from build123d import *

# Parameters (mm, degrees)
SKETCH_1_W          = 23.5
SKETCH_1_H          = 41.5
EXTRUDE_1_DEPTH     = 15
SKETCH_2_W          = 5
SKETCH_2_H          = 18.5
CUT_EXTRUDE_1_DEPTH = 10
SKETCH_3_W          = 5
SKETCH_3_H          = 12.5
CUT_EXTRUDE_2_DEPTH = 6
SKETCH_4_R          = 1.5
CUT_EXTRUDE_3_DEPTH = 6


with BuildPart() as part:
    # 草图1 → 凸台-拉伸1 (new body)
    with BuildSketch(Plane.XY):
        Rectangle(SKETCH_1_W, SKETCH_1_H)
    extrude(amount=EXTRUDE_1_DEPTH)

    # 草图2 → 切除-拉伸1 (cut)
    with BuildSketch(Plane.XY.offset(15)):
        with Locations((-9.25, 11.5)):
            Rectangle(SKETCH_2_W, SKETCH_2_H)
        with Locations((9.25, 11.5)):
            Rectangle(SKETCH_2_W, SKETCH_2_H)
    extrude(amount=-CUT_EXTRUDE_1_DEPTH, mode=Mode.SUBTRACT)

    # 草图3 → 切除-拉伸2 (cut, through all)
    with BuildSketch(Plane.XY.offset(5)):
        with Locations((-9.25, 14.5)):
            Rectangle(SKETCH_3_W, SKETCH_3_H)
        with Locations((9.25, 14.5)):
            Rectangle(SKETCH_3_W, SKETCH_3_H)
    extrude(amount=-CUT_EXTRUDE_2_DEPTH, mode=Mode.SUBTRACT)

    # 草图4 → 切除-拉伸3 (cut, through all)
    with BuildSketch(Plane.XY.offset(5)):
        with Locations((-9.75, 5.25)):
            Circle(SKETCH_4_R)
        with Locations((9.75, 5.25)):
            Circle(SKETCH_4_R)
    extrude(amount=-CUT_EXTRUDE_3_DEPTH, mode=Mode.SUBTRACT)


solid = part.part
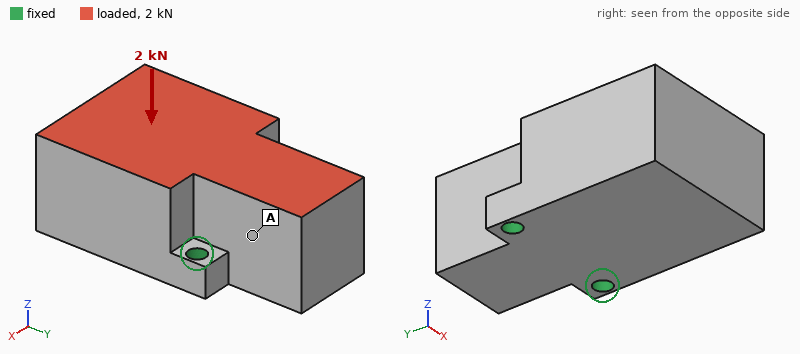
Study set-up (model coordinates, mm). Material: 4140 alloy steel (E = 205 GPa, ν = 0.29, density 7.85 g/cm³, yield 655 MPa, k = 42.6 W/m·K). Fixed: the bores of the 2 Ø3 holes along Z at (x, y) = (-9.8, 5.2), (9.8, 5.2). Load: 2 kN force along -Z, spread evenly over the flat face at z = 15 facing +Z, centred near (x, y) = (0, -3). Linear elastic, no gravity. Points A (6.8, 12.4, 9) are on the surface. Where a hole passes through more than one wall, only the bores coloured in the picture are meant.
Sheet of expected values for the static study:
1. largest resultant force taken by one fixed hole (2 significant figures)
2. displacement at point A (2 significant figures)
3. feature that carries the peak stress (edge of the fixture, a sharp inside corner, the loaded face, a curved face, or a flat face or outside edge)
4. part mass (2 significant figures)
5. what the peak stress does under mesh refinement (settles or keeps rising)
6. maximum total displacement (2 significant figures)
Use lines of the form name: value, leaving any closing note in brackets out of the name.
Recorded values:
largest resultant force taken by one fixed hole: 1.0 kN
displacement at point A: 10 µm
feature that carries the peak stress: edge of the fixture
part mass: 95 g
what the peak stress does under mesh refinement: keeps rising
maximum total displacement: 35 µm
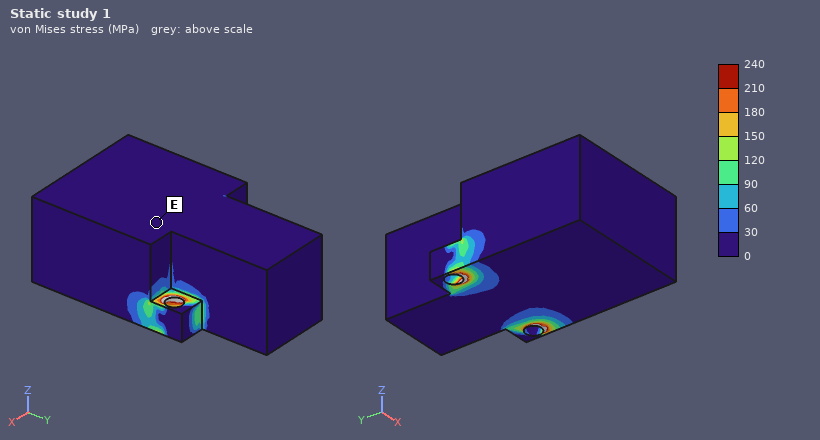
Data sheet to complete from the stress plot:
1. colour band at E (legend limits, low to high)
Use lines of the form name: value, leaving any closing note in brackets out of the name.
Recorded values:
colour band at E: 0 to 30 MPa
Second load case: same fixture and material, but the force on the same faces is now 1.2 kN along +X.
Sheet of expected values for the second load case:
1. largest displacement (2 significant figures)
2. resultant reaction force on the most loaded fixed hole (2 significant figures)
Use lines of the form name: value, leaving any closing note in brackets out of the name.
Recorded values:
largest displacement: 4.3 µm
resultant reaction force on the most loaded fixed hole: 1.1 kN
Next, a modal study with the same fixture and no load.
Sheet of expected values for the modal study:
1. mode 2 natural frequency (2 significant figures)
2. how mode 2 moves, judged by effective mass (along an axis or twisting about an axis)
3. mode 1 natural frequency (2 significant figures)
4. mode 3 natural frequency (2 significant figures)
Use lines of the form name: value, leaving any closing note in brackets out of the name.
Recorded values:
mode 2 natural frequency: 13 kHz
how mode 2 moves, judged by effective mass: along X
mode 1 natural frequency: 3800 Hz
mode 3 natural frequency: 17 kHz
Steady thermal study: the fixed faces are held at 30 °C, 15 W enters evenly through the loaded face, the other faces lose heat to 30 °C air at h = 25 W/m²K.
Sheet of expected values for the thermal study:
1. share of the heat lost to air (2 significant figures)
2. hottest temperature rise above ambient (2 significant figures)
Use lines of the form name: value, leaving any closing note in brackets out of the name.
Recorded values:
share of the heat lost to air: 8.1 %
hottest temperature rise above ambient: 24 K
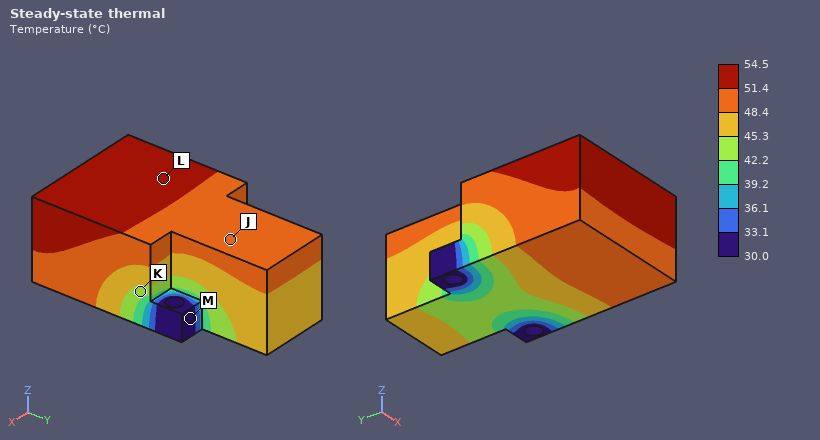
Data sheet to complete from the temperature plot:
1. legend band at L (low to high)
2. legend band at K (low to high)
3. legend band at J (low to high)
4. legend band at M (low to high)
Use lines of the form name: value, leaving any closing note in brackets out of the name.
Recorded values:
legend band at L: 51.4 to 54.5 °C
legend band at K: 42.2 to 45.3 °C
legend band at J: 48.4 to 51.4 °C
legend band at M: 30.0 to 33.1 °C
